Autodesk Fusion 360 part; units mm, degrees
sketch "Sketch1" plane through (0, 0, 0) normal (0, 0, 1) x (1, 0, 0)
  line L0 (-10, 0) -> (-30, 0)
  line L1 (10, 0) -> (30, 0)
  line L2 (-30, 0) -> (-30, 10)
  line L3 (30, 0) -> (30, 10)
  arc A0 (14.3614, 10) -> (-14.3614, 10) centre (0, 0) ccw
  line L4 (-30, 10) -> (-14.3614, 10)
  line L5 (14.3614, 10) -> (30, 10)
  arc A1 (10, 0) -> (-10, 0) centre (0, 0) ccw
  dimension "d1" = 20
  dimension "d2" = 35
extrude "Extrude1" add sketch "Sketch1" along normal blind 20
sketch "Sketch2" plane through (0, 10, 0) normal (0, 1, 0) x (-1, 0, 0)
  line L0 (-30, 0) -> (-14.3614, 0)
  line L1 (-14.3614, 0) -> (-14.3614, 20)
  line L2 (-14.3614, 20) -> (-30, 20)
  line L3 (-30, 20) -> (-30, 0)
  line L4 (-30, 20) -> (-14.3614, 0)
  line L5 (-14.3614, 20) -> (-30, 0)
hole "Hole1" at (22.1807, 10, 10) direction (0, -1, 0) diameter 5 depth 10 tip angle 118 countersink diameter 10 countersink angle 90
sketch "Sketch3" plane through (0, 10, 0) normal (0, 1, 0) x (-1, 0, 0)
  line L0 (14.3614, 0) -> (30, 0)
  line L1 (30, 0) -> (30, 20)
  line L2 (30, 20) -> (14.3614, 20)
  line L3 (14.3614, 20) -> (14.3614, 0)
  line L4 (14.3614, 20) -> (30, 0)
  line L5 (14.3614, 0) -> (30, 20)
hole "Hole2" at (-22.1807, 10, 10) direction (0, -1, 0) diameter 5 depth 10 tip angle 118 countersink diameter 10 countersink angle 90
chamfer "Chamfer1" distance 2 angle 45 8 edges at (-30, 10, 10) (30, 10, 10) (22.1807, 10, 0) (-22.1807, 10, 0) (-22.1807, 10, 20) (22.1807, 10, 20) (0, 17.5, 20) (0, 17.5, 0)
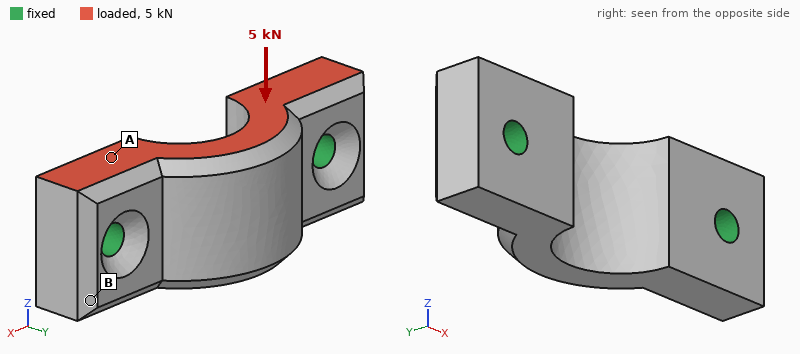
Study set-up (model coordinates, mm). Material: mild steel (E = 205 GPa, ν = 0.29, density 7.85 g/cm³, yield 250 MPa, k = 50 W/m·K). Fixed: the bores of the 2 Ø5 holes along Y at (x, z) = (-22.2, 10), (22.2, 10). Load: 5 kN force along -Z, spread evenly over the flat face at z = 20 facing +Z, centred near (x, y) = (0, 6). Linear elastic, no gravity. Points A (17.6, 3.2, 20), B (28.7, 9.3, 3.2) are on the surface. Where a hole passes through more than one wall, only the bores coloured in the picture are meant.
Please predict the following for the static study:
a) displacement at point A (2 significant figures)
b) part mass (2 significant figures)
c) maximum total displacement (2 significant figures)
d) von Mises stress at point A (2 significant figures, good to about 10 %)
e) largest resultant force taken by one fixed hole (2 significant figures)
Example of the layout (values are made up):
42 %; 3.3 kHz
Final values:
2.6 µm; 87 g; 7.4 µm; 18 MPa; 2.5 kN
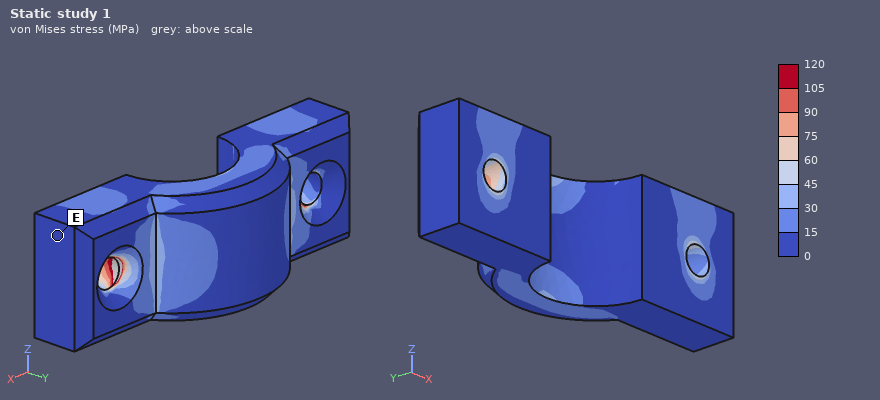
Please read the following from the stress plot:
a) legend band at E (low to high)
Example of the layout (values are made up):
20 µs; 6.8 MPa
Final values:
0 to 15 MPa
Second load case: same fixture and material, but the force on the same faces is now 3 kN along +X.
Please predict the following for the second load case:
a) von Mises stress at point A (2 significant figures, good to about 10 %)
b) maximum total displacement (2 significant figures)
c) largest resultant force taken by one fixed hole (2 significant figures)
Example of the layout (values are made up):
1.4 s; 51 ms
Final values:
13 MPa; 2.4 µm; 1.6 kN
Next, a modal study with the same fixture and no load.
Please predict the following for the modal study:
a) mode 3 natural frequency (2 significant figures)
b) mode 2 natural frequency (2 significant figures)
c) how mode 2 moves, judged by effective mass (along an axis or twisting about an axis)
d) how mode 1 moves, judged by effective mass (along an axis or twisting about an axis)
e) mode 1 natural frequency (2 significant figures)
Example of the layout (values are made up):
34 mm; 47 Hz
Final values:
30 kHz; 23 kHz; along Y; along Z; 15 kHz
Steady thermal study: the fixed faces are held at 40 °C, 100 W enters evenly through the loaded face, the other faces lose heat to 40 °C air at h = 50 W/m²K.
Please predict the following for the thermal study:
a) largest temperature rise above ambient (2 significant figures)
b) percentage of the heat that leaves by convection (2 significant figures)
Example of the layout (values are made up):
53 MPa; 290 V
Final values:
73 K; 5.2 %
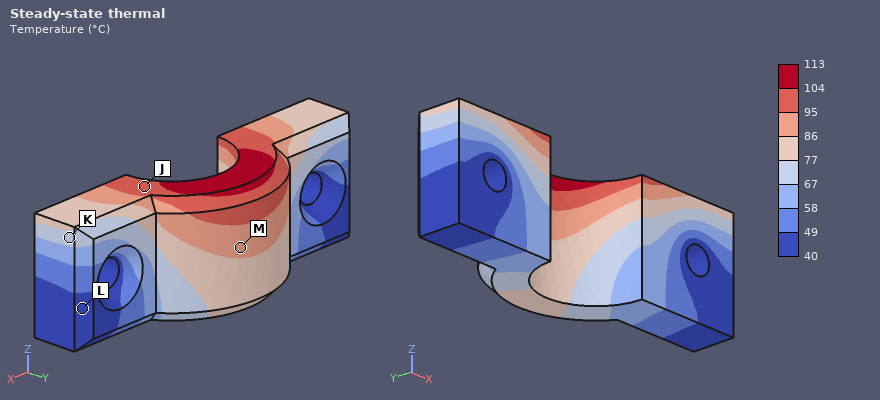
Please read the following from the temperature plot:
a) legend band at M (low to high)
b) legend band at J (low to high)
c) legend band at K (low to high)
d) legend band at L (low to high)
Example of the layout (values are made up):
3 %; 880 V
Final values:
86 to 95 °C; 95 to 104 °C; 67 to 77 °C; 40 to 49 °C
